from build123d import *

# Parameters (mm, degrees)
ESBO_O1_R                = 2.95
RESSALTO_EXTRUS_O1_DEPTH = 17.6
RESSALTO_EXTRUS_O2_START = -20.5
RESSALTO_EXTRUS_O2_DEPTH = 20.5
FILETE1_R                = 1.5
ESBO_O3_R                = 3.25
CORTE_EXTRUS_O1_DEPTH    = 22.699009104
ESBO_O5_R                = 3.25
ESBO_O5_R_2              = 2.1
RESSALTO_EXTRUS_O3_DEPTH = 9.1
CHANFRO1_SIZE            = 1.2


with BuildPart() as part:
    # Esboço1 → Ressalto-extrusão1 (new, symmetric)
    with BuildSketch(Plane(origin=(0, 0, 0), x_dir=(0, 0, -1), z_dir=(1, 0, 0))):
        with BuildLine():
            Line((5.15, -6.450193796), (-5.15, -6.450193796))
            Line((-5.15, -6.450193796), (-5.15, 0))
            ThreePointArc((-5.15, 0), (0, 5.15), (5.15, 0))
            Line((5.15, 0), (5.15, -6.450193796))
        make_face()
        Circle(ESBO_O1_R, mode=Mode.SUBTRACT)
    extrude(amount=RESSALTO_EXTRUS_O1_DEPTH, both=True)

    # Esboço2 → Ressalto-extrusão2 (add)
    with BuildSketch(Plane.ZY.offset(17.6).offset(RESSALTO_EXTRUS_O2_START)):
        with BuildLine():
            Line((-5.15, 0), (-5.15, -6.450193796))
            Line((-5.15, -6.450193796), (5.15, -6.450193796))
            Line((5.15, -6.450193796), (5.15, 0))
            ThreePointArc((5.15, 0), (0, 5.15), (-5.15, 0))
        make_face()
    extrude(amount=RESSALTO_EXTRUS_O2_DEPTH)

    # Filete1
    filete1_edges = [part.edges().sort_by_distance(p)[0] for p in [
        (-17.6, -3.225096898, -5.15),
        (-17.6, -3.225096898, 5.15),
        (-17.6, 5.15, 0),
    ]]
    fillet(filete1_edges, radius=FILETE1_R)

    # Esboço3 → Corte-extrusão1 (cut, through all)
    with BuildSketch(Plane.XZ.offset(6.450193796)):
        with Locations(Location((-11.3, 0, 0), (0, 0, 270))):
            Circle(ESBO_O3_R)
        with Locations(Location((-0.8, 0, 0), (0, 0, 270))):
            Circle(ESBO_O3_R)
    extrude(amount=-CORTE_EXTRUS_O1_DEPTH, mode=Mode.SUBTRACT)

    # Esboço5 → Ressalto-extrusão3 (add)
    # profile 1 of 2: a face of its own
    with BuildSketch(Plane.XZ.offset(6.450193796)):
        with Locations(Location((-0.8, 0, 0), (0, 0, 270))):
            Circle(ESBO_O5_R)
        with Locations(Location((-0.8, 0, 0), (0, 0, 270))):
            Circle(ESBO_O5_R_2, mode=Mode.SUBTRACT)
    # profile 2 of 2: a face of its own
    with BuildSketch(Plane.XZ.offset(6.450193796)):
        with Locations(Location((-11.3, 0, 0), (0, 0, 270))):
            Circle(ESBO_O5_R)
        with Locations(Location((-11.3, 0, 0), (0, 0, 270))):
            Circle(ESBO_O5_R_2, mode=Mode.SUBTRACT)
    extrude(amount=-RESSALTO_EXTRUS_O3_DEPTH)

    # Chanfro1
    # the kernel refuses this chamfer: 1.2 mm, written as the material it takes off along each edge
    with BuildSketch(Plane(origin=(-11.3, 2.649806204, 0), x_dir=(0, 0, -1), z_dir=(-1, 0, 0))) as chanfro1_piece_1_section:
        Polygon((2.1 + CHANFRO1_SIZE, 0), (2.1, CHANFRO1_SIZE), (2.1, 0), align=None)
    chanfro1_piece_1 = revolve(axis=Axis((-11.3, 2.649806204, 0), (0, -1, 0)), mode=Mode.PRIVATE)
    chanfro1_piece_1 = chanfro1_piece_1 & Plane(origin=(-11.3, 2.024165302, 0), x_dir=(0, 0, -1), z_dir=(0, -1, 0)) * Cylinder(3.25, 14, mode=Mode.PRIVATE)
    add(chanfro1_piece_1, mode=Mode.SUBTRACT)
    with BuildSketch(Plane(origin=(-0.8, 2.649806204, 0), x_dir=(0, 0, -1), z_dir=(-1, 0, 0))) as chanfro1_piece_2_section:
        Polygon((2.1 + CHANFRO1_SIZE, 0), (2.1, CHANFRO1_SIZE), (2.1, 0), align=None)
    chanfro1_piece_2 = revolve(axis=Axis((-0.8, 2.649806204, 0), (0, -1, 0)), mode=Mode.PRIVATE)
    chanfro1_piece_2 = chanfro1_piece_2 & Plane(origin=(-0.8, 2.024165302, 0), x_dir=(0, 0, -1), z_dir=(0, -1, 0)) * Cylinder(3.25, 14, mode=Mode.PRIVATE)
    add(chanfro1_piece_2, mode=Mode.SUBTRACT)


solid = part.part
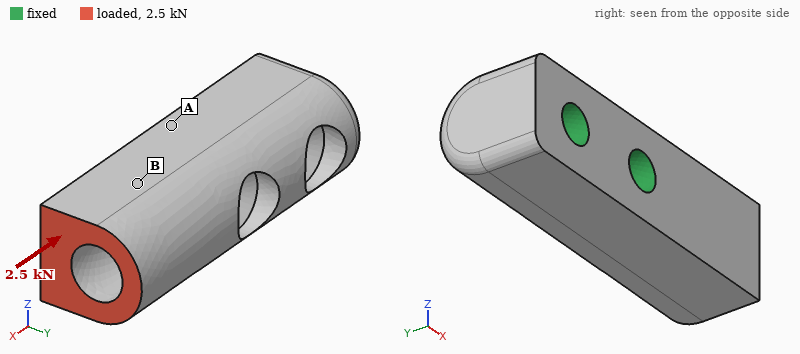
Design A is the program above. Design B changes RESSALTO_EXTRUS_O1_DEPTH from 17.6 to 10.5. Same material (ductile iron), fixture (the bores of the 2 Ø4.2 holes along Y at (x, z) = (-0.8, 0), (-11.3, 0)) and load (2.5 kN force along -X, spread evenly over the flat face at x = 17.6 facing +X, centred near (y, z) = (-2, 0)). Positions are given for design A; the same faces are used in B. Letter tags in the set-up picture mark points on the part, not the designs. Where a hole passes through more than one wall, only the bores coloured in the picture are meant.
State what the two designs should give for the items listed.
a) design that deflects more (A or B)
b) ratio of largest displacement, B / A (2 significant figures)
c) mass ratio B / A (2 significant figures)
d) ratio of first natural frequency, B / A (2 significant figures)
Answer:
A
0.74
0.81
2.1
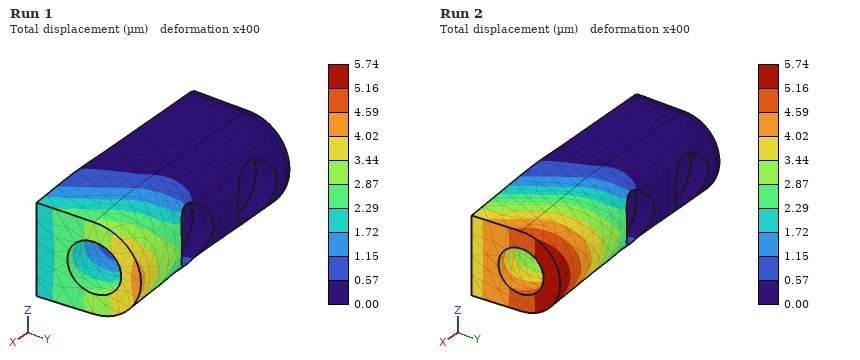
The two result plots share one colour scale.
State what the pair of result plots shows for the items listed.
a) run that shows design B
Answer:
Run 1
